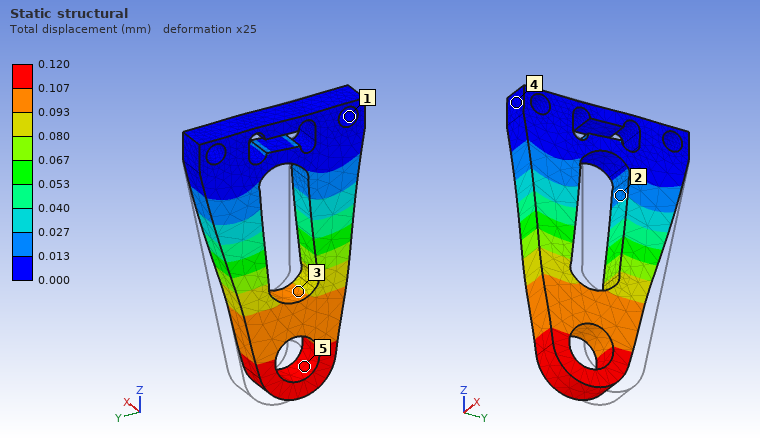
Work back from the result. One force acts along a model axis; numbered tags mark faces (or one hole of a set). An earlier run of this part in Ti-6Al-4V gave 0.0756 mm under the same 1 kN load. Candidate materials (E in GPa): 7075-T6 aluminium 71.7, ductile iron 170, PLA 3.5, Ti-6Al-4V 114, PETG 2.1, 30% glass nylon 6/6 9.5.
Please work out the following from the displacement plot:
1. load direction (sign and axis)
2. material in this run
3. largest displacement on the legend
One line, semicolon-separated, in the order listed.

-Y; 7075-T6 aluminium; 0.120 mm
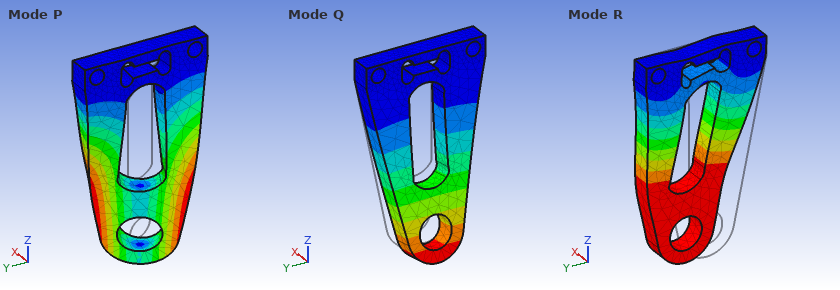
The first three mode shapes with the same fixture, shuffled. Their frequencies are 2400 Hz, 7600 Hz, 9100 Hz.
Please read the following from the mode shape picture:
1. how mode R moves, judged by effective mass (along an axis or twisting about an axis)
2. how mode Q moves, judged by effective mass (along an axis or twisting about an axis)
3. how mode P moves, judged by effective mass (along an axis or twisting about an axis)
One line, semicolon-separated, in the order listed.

along Y; along X; twisting about Z
